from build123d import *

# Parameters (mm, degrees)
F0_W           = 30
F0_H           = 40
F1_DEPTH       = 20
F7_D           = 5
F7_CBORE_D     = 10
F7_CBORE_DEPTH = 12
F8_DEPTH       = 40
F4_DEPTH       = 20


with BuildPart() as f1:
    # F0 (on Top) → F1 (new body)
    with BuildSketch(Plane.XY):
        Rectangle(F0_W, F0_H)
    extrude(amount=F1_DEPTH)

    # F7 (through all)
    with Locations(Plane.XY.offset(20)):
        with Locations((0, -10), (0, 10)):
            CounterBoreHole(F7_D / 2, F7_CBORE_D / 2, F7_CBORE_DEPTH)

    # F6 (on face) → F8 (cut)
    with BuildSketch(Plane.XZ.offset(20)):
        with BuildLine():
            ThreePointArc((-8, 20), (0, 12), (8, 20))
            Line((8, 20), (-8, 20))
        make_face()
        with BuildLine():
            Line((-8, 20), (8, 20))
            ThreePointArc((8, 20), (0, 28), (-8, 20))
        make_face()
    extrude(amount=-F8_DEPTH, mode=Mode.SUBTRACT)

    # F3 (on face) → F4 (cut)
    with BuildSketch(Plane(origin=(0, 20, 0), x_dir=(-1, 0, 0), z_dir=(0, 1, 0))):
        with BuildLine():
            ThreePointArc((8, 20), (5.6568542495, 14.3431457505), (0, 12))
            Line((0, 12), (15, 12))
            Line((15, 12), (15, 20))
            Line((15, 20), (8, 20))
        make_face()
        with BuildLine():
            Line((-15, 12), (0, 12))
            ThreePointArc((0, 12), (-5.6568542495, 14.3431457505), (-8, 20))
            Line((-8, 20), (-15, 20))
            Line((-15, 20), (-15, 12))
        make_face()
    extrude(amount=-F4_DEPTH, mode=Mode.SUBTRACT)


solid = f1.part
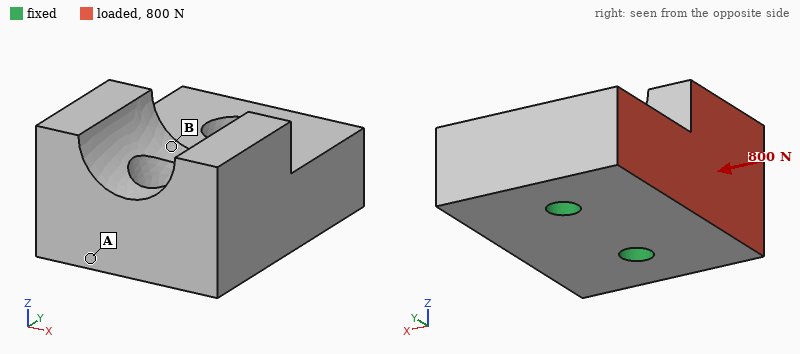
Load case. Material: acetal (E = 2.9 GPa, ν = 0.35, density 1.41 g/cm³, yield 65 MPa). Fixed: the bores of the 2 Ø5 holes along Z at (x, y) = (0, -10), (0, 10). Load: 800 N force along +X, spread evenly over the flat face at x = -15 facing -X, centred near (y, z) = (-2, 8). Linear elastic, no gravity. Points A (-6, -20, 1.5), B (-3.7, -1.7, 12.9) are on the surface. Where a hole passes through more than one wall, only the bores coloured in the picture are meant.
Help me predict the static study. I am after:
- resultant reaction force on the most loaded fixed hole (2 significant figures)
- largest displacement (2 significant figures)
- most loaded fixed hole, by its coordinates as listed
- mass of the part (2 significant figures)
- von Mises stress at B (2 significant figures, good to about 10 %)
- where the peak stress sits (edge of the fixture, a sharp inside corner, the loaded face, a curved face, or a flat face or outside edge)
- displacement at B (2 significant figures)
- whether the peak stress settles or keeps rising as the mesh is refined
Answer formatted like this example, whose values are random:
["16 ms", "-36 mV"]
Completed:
["490 N", "0.11 mm", "(0, -10)", "23 g", "6.9 MPa", "edge of the fixture", "0.036 mm", "keeps rising"]
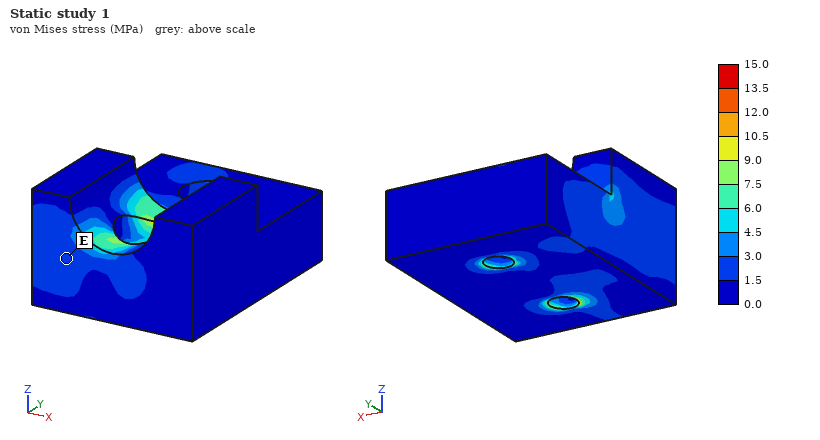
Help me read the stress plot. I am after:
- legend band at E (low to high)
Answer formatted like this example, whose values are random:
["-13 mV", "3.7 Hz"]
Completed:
["1.5 to 3.0 MPa"]
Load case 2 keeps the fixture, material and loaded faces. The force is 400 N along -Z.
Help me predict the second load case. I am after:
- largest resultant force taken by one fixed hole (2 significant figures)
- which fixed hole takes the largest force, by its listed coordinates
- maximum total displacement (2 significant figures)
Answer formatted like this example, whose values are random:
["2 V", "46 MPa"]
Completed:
["240 N", "(0, -10)", "0.13 mm"]
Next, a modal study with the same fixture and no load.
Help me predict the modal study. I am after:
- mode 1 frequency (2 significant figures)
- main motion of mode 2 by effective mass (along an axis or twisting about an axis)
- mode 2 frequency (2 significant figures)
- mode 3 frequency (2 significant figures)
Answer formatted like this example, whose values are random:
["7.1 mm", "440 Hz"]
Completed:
["3700 Hz", "along Z", "6000 Hz", "6800 Hz"]
